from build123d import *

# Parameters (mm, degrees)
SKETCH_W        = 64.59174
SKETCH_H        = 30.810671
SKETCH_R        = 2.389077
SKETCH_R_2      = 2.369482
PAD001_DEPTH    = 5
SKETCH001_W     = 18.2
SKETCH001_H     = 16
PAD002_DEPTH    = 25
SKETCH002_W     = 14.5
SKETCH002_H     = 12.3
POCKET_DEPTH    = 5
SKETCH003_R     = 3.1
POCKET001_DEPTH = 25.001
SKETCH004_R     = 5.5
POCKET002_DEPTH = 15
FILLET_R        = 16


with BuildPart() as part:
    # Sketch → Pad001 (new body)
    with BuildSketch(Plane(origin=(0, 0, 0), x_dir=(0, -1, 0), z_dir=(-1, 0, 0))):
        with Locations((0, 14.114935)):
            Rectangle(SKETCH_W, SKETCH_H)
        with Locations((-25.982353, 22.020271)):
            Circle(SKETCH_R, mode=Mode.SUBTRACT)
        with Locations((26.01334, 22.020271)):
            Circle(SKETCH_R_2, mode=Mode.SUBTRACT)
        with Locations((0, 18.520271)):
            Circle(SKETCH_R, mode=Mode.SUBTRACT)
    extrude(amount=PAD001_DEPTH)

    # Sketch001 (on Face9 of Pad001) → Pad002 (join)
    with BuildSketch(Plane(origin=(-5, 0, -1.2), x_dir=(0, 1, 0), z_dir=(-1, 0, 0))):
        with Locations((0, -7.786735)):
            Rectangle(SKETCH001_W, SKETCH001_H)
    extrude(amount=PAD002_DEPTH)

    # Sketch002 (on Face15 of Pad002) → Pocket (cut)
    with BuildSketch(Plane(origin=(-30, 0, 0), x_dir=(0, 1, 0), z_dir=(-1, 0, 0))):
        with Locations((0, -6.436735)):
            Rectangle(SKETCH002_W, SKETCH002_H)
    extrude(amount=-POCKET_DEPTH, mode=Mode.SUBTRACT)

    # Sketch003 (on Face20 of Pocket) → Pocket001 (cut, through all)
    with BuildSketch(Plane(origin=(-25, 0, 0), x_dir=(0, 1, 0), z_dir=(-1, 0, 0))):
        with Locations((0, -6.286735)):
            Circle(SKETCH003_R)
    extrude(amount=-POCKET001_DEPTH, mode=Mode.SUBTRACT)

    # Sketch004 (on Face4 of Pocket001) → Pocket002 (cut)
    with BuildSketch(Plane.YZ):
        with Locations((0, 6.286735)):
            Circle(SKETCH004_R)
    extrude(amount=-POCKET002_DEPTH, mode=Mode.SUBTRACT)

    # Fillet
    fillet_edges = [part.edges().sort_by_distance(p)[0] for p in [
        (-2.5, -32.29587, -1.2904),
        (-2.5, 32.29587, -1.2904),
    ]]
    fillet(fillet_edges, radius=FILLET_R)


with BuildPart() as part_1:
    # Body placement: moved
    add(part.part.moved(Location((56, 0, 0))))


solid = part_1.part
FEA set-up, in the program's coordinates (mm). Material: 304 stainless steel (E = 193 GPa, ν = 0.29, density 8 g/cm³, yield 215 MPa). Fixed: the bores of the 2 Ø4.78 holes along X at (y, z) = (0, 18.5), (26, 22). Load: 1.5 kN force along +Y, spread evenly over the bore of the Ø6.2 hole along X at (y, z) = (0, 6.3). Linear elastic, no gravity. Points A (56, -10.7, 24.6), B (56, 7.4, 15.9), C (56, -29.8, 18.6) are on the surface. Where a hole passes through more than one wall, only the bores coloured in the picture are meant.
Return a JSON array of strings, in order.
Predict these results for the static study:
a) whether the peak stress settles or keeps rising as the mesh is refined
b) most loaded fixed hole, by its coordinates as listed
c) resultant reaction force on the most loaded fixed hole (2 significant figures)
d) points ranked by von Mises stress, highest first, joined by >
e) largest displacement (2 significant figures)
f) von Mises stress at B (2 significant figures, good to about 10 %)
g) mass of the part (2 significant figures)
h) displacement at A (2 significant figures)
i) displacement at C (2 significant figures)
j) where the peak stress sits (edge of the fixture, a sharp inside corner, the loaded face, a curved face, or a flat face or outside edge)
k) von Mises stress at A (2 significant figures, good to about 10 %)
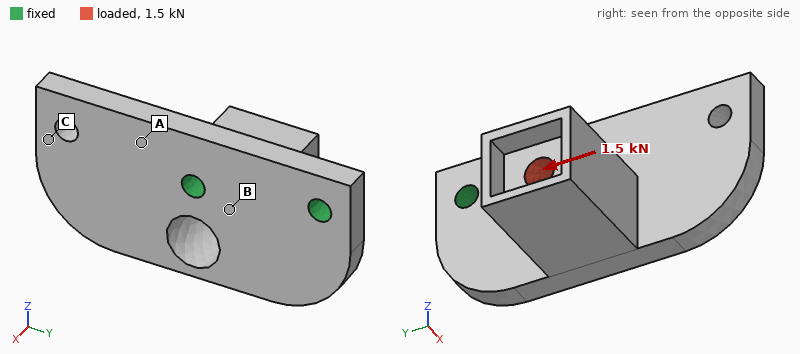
["keeps rising", "(0, 18.5)", "1.3 kN", "B > A > C", "43 µm", "44 MPa", "110 g", "6.6 µm", "29 µm", "edge of the fixture", "28 MPa"]
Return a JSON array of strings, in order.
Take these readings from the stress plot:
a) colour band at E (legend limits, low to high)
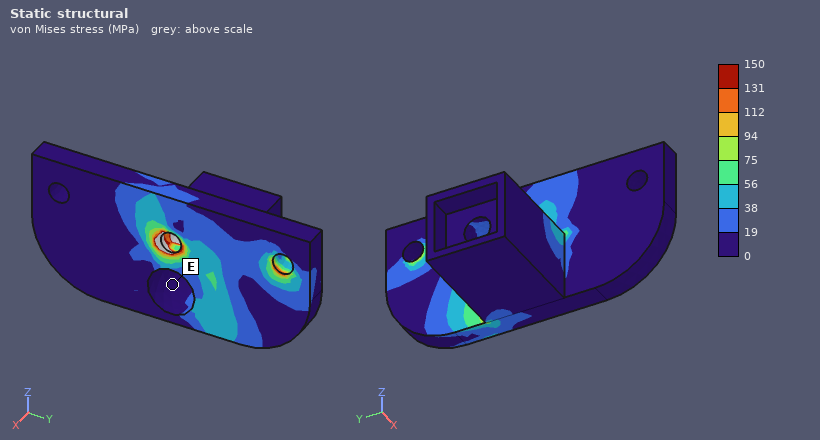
["0 to 19 MPa"]
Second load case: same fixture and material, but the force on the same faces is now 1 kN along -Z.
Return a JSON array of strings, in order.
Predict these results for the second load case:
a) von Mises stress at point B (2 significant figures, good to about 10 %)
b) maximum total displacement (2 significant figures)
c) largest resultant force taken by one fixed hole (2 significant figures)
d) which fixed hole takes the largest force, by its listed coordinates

["73 MPa", "71 µm", "980 N", "(0, 18.5)"]
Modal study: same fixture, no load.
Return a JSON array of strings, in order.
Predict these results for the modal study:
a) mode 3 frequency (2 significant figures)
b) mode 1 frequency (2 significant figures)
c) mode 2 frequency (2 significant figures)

["7200 Hz", "3400 Hz", "4200 Hz"]
